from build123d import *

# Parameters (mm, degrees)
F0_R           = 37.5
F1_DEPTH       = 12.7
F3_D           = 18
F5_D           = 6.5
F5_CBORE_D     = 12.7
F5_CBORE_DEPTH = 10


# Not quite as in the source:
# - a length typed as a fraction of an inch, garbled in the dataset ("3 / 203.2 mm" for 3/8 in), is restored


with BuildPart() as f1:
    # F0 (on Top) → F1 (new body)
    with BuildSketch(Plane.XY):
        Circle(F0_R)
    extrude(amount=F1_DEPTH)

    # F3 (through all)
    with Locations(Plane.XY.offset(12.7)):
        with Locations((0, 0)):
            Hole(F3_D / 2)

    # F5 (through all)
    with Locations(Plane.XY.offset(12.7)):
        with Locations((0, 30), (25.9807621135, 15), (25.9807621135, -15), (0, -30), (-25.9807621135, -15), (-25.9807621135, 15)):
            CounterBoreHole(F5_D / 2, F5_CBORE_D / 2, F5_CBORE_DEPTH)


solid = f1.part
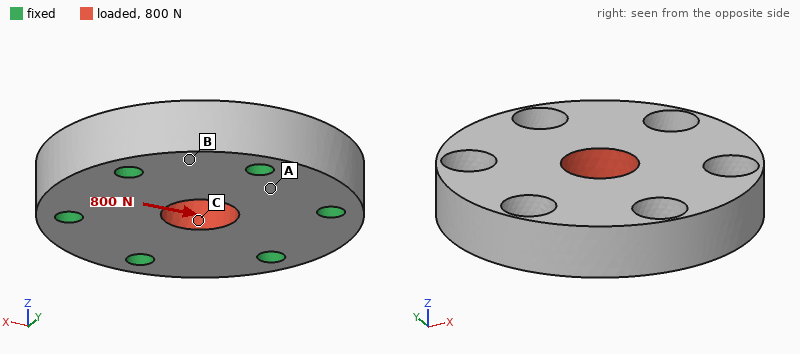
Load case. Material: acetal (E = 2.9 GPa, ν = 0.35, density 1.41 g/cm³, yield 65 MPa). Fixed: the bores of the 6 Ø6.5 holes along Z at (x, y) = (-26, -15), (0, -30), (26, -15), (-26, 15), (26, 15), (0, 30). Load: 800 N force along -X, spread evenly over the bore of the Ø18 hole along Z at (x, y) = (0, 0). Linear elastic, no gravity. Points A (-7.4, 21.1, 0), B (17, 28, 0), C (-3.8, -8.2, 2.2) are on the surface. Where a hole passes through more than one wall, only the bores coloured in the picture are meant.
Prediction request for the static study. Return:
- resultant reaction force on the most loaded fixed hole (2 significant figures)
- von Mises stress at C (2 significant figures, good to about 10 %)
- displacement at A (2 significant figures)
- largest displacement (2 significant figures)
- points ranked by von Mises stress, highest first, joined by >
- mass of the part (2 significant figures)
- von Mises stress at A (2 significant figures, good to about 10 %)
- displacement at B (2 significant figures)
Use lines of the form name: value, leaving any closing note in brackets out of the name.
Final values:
resultant reaction force on the most loaded fixed hole: 160 N
von Mises stress at C: 1.8 MPa
displacement at A: 6.6 µm
largest displacement: 19 µm
points ranked by von Mises stress, highest first, joined by >: C > A > B
mass of the part: 63 g
von Mises stress at A: 0.89 MPa
displacement at B: 5.6 µm
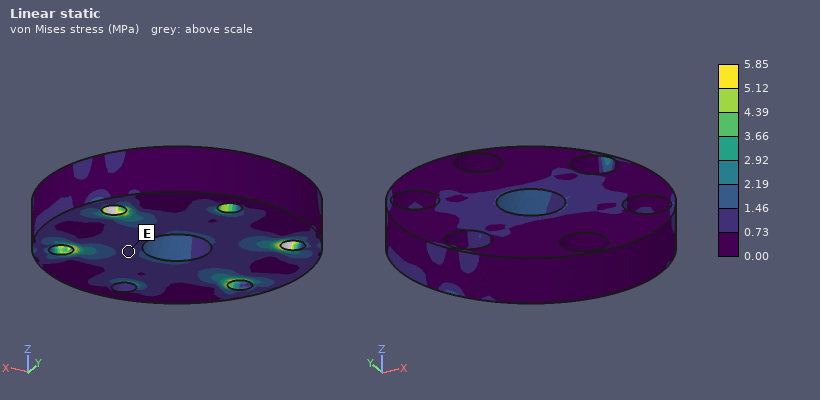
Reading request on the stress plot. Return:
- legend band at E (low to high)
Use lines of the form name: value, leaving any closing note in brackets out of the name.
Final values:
legend band at E: 0.73 to 1.46 MPa
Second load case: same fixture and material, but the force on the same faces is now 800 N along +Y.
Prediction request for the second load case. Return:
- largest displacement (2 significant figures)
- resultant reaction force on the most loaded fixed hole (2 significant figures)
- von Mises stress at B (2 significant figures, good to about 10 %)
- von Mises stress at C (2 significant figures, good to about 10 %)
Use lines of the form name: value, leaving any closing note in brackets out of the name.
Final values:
largest displacement: 19 µm
resultant reaction force on the most loaded fixed hole: 180 N
von Mises stress at B: 0.54 MPa
von Mises stress at C: 1.2 MPa
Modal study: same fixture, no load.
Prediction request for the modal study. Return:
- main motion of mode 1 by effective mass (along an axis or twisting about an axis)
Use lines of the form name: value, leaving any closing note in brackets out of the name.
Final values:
main motion of mode 1 by effective mass: along Z
